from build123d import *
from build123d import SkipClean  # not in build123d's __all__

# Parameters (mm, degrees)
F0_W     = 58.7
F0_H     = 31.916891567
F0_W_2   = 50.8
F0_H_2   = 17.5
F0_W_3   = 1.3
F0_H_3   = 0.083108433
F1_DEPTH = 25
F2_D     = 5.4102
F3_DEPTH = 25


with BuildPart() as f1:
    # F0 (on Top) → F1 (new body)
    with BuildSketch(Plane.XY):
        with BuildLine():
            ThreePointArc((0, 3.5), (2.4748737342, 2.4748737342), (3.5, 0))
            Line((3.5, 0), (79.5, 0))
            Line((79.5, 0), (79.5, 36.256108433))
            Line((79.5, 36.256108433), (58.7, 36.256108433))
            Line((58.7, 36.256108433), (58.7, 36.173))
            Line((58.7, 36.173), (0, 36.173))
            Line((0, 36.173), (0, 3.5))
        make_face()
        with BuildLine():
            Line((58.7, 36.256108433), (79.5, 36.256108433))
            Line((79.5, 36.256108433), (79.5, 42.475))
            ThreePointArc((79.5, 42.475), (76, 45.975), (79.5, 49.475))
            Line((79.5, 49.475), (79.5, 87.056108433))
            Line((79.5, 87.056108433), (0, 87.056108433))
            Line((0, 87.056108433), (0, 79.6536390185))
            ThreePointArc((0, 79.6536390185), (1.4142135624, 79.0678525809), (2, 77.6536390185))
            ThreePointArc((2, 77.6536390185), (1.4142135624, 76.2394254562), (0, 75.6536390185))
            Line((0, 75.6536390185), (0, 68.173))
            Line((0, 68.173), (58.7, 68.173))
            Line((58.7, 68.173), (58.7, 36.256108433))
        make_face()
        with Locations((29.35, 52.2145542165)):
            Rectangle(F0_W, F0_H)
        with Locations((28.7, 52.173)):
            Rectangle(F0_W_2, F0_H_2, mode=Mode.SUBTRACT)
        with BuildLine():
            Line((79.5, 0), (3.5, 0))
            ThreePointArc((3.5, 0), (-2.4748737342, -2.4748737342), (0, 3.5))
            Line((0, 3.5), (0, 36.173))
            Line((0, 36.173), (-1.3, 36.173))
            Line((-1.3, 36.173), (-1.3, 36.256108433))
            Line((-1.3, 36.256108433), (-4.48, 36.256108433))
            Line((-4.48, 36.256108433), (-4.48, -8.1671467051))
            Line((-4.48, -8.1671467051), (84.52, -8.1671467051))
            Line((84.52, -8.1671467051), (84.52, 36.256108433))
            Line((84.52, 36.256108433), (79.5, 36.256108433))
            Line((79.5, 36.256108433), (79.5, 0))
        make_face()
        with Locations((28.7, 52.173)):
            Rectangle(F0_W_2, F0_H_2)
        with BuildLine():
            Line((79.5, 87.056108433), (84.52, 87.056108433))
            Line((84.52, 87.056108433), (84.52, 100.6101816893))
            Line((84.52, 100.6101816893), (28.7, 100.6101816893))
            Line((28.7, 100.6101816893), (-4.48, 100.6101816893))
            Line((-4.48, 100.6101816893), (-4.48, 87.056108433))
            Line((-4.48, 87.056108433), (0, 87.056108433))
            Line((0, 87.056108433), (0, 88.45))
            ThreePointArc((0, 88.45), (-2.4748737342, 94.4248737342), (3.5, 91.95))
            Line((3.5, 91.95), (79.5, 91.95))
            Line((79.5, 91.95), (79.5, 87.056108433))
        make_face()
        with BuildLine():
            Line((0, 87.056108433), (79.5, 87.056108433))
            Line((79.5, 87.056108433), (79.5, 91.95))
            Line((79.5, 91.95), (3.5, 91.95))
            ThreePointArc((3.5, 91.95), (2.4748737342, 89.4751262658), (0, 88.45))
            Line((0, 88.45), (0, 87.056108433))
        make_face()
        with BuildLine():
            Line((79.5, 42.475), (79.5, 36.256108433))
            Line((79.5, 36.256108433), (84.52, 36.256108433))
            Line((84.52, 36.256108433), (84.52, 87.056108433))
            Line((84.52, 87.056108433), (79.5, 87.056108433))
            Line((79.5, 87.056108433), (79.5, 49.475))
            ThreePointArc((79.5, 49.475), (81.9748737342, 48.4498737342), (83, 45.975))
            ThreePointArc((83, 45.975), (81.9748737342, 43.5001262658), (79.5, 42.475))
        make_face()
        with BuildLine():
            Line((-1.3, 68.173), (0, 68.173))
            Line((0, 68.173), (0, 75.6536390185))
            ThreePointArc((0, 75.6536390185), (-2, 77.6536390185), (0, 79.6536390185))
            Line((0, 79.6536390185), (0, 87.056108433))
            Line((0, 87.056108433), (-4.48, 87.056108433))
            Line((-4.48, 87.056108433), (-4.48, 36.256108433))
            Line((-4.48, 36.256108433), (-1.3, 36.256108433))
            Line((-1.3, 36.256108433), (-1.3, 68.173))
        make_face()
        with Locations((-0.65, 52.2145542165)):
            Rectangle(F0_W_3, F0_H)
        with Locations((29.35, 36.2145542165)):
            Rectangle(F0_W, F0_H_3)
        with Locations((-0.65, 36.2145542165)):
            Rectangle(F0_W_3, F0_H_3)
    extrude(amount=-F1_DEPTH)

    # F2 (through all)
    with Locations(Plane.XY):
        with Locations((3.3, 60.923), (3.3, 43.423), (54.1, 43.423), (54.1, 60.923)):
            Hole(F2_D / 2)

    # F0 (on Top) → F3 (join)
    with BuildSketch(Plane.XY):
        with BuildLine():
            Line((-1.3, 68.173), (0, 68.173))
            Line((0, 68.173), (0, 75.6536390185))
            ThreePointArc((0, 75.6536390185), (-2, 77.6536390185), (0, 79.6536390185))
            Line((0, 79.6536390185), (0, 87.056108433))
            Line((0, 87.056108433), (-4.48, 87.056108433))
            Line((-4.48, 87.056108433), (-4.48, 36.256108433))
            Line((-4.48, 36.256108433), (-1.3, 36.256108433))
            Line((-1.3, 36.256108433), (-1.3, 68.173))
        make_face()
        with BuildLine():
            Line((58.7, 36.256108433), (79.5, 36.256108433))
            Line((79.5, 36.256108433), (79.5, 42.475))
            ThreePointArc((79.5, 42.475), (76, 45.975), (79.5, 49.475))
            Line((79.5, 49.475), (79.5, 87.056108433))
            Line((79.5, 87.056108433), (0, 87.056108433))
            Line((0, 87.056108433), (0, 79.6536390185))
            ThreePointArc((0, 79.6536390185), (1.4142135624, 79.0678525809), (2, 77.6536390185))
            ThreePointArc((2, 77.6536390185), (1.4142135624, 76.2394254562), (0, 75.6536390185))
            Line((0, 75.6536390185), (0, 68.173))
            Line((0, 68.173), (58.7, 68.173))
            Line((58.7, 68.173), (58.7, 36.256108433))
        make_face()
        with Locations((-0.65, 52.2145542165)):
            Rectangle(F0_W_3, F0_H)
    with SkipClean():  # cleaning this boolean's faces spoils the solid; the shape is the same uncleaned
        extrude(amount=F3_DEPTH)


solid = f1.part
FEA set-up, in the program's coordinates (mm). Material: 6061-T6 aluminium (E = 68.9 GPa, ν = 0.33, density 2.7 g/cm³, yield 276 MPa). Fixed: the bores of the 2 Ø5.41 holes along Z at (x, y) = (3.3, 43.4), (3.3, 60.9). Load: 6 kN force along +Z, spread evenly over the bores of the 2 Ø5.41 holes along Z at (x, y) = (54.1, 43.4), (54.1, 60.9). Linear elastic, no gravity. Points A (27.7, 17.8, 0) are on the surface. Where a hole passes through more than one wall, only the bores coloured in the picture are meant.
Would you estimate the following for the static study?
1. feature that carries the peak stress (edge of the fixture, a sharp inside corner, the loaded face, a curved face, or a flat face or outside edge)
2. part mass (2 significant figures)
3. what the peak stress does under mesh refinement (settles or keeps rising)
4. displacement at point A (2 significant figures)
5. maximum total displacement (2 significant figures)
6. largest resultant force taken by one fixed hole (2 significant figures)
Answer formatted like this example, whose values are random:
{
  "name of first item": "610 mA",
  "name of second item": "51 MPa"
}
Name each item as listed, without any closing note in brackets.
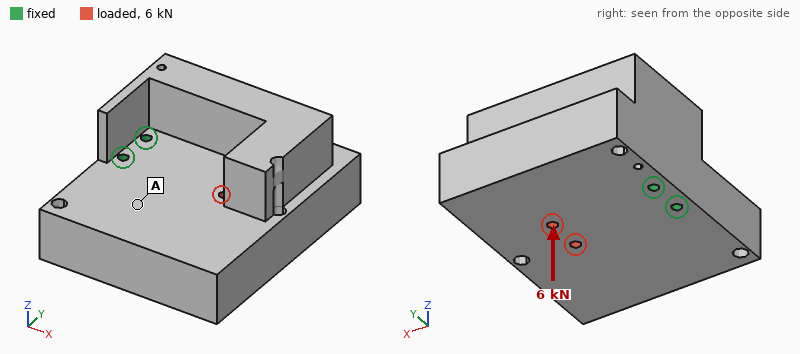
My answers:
{
  "feature that carries the peak stress": "edge of the fixture",
  "part mass": "800 g",
  "what the peak stress does under mesh refinement": "keeps rising",
  "displacement at point A": "0.030 mm",
  "maximum total displacement": "0.11 mm",
  "largest resultant force taken by one fixed hole": "3.1 kN"
}
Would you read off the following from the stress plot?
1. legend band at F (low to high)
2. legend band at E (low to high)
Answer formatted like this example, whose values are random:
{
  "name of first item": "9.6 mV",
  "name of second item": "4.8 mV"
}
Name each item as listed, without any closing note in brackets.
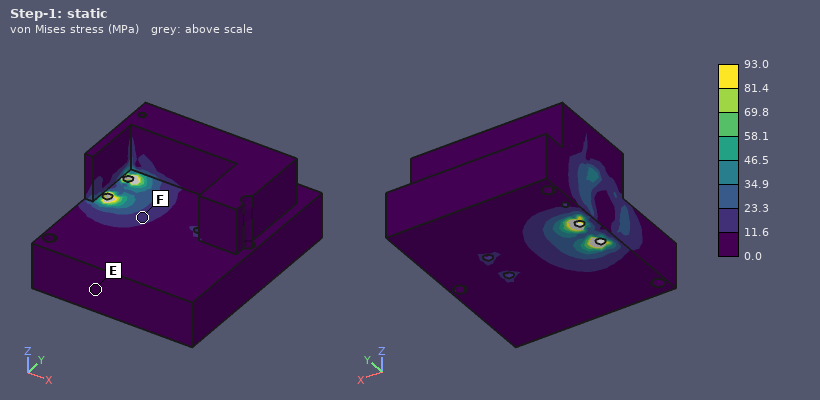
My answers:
{
  "legend band at F": "11.6 to 23.3 MPa",
  "legend band at E": "0.0 to 11.6 MPa"
}
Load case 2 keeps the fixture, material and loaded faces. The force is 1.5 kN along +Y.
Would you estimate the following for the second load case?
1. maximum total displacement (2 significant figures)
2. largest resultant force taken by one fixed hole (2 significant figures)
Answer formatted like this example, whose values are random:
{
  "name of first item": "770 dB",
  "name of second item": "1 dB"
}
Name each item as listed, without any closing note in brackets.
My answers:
{
  "maximum total displacement": "21 µm",
  "largest resultant force taken by one fixed hole": "3.4 kN"
}
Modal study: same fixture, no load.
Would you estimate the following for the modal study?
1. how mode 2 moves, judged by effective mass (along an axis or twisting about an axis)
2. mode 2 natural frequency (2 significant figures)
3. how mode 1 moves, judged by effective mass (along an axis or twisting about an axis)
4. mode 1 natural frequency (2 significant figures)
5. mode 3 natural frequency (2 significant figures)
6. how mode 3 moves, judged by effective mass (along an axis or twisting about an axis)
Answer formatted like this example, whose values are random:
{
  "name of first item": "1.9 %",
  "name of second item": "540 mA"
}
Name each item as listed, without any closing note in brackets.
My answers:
{
  "how mode 2 moves, judged by effective mass": "along Y",
  "mode 2 natural frequency": "2000 Hz",
  "how mode 1 moves, judged by effective mass": "along Z",
  "mode 1 natural frequency": "1900 Hz",
  "mode 3 natural frequency": "3000 Hz",
  "how mode 3 moves, judged by effective mass": "twisting about X"
}
